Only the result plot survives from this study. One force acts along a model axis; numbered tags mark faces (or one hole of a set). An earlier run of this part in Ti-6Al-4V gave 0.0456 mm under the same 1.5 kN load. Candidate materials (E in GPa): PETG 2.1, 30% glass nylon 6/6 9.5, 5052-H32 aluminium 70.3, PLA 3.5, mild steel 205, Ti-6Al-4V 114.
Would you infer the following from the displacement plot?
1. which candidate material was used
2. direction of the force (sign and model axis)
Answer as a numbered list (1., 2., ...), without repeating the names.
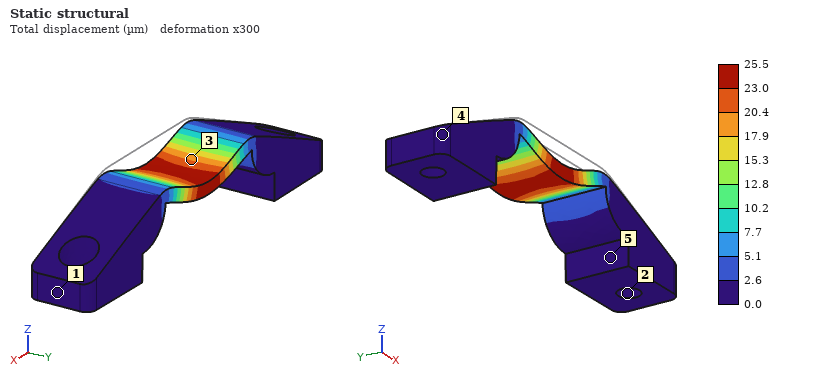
1. mild steel
2. -Z
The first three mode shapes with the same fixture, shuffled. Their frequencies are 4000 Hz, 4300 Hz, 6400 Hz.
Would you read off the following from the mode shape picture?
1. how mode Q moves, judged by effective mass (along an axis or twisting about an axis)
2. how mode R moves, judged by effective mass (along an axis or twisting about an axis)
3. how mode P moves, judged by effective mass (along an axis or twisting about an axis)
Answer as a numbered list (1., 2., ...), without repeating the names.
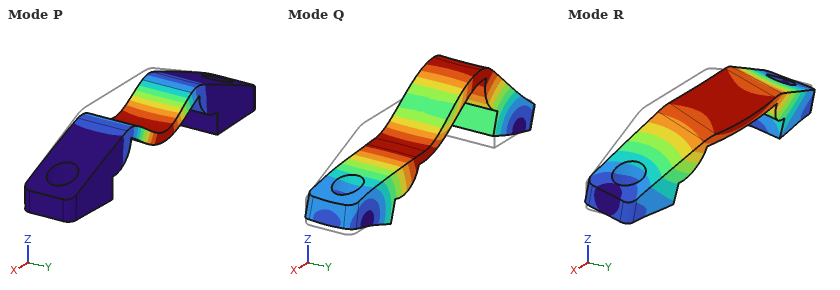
1. along X
2. along Y
3. along Z
